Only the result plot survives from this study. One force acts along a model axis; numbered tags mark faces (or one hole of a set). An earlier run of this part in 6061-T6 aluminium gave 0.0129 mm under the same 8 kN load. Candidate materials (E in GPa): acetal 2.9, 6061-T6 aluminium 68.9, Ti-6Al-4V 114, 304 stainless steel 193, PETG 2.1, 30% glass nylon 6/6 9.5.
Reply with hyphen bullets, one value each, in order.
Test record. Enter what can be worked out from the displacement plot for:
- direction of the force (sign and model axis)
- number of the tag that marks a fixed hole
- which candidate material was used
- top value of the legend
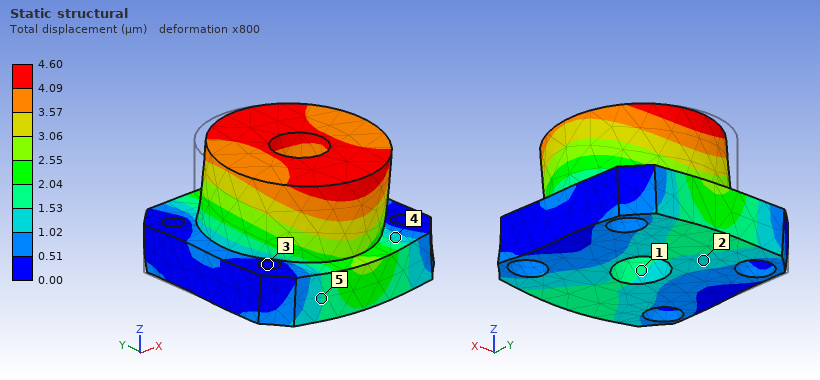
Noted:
- -Y
- 3
- 304 stainless steel
- 4.60 µm
